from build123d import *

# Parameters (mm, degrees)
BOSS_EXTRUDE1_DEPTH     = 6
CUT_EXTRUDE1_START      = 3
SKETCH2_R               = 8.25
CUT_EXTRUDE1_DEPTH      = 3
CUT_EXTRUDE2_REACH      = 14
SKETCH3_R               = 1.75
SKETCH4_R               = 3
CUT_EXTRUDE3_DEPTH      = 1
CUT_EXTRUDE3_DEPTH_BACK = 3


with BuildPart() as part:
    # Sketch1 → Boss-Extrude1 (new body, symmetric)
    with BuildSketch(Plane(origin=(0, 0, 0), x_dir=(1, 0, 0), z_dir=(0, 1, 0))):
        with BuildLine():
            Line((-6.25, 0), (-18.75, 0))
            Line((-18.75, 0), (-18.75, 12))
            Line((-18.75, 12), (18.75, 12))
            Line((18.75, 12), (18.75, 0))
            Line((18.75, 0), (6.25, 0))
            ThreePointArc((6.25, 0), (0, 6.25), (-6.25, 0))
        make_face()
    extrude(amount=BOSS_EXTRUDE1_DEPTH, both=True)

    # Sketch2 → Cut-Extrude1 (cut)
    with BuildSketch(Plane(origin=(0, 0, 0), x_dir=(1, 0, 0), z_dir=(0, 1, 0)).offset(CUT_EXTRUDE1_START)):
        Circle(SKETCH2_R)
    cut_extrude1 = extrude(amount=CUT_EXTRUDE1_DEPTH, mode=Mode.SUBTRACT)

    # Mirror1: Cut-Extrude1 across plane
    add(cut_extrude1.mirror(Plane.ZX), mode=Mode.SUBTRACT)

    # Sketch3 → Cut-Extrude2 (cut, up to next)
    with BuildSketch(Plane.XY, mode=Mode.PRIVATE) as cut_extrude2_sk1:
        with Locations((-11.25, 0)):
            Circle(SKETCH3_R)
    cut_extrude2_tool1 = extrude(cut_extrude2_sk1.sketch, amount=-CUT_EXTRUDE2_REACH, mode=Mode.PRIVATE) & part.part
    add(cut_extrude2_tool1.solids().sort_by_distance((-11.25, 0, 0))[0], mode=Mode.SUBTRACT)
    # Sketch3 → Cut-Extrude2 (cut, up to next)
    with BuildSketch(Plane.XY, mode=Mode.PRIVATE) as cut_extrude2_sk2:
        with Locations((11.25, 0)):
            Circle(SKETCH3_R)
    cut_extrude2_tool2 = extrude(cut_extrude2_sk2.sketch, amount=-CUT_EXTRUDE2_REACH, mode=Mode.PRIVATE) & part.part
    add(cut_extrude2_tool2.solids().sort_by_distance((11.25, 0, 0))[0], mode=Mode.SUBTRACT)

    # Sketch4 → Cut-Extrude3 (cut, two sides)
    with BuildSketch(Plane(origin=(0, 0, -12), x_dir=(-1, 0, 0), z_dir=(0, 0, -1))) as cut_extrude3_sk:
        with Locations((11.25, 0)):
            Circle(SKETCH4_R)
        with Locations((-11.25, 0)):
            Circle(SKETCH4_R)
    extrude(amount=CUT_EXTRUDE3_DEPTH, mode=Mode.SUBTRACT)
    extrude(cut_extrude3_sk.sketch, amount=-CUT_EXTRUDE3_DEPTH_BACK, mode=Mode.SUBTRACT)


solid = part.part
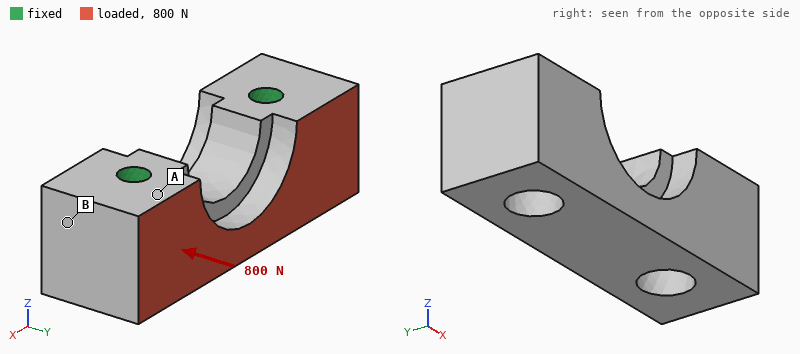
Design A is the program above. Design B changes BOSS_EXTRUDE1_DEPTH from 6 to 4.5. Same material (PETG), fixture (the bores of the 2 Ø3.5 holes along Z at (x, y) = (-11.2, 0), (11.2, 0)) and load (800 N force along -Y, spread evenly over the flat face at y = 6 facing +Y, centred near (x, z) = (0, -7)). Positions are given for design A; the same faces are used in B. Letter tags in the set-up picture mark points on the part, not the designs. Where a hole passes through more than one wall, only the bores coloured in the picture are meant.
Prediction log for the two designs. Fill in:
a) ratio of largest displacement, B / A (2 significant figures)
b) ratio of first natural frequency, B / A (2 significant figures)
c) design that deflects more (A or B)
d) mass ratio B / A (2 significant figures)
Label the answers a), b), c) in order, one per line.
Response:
a) 1.3
b) 1.1
c) B
d) 0.75
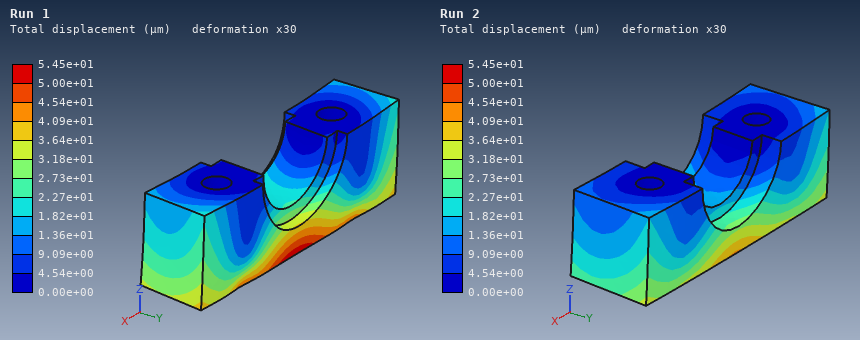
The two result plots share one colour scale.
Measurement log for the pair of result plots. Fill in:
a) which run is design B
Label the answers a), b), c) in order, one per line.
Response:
a) Run 1
